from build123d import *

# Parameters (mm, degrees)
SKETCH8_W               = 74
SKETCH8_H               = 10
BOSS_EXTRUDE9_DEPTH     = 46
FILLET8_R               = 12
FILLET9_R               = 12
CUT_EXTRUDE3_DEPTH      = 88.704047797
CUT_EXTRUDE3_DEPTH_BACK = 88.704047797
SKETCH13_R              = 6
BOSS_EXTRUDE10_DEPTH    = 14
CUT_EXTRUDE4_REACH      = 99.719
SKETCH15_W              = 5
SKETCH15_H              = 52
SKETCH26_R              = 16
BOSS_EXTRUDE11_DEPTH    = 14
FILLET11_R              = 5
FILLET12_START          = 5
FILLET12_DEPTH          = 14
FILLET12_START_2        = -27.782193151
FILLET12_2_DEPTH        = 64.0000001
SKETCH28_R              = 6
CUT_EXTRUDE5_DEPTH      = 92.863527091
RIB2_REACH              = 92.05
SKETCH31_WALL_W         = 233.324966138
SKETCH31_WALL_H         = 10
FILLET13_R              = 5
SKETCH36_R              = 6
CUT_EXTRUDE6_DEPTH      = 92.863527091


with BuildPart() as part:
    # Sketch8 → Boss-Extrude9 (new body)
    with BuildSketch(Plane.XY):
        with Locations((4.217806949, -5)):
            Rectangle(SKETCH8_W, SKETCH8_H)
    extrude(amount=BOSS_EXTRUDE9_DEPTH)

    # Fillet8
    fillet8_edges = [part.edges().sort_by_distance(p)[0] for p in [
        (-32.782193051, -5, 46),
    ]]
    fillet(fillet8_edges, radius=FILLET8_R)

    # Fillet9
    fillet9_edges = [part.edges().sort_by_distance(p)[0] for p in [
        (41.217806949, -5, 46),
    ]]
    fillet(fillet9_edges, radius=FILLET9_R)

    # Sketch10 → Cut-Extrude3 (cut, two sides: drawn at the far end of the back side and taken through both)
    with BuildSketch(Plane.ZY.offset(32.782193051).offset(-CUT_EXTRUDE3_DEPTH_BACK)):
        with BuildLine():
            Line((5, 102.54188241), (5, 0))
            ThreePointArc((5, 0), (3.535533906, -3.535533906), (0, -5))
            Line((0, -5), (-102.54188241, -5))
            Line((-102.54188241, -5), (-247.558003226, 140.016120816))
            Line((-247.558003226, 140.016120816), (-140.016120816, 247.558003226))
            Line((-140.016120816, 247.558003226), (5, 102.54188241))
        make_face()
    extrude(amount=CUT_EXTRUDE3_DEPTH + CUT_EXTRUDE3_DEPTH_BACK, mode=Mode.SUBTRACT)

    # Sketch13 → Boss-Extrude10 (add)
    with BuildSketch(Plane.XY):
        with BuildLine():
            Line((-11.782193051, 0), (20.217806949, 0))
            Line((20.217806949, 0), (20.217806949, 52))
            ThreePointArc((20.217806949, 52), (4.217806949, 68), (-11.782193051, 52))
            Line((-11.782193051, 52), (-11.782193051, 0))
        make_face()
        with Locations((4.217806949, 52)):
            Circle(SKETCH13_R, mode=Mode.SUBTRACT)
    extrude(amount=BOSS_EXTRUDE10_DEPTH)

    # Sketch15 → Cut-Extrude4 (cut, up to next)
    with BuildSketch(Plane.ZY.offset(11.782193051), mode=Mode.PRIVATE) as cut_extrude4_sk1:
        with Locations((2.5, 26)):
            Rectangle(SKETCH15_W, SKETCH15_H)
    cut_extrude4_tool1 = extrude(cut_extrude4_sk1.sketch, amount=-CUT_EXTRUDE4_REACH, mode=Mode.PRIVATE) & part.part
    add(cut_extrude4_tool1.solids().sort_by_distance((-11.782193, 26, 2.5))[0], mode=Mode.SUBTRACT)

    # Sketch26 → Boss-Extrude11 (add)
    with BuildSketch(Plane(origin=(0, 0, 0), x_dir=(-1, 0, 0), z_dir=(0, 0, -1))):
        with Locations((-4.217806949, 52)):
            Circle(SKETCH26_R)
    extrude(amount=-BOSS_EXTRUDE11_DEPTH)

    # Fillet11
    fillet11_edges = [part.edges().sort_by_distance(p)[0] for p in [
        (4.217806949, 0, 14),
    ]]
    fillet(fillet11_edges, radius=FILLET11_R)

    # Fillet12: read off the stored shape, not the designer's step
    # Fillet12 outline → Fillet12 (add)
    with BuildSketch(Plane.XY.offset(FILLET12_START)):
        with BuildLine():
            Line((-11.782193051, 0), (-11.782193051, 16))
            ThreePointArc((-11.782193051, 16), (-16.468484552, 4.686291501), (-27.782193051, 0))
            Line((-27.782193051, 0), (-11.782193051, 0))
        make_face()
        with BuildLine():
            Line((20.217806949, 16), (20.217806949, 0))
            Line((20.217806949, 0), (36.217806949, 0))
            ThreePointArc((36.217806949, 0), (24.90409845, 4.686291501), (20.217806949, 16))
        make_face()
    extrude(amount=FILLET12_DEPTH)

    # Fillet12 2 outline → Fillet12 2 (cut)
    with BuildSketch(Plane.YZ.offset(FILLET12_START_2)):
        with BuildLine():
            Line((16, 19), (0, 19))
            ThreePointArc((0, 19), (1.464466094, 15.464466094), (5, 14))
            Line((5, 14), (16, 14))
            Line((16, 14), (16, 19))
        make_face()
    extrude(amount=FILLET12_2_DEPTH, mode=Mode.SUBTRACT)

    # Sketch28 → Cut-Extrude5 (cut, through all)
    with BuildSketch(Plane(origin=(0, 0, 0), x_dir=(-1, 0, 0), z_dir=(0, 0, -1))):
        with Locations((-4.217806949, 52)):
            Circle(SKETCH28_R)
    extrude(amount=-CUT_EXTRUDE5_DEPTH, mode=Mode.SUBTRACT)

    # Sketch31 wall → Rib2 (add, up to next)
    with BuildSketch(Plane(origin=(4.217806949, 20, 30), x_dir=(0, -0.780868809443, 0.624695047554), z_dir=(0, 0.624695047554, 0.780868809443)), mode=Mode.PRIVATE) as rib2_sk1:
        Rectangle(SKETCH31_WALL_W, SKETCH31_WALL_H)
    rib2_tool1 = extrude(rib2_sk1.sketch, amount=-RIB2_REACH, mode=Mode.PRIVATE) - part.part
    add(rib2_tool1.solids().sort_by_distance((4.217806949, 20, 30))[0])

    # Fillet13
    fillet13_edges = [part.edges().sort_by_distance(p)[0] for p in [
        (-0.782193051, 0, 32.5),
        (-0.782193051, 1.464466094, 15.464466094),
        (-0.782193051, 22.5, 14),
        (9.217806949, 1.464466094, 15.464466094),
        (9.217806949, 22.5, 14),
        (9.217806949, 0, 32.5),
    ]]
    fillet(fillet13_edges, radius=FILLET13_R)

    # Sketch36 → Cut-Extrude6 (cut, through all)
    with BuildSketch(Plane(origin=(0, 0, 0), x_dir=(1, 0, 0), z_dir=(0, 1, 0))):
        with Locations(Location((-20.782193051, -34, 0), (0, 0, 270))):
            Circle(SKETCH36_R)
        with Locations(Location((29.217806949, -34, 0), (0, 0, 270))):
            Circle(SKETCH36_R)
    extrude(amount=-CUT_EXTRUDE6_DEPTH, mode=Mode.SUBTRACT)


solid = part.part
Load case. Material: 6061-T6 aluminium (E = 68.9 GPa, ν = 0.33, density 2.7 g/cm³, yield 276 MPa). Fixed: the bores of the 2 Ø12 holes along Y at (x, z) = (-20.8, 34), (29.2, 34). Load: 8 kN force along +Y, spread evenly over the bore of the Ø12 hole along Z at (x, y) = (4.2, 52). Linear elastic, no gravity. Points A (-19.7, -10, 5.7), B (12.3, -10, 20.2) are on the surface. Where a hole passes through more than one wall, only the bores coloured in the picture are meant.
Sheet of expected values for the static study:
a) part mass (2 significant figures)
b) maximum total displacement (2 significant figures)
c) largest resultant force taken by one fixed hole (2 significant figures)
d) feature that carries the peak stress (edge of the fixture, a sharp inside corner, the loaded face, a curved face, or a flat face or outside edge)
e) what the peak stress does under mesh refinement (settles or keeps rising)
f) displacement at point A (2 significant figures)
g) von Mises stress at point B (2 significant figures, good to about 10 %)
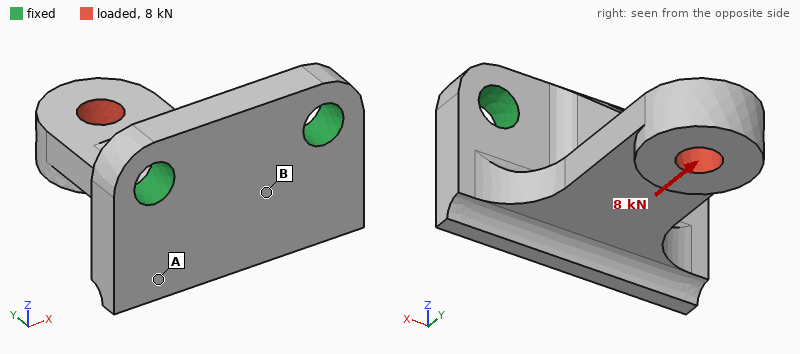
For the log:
160 g
0.40 mm
4.1 kN
edge of the fixture
keeps rising
0.095 mm
37 MPa
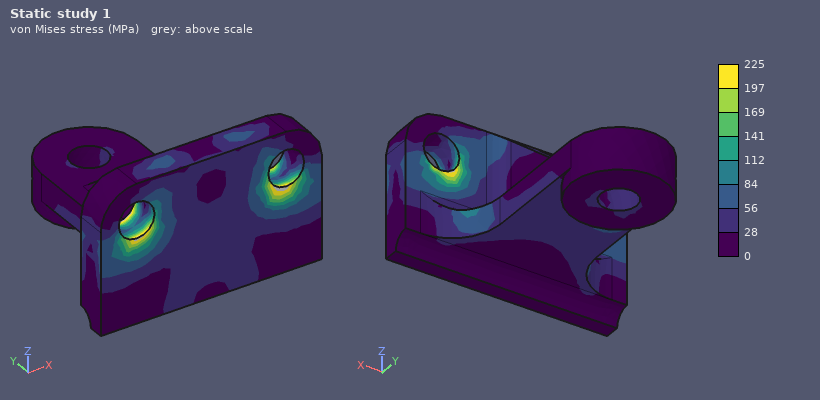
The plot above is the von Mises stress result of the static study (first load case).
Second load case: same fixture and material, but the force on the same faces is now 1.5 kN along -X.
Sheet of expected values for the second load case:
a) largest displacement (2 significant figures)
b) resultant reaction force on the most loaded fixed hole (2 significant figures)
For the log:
0.11 mm
2.2 kN
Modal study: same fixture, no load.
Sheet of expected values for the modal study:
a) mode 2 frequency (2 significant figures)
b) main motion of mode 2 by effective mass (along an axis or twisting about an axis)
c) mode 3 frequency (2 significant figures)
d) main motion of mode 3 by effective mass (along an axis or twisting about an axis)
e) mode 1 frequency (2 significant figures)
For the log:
3600 Hz
along X
6800 Hz
along Y
2400 Hz
